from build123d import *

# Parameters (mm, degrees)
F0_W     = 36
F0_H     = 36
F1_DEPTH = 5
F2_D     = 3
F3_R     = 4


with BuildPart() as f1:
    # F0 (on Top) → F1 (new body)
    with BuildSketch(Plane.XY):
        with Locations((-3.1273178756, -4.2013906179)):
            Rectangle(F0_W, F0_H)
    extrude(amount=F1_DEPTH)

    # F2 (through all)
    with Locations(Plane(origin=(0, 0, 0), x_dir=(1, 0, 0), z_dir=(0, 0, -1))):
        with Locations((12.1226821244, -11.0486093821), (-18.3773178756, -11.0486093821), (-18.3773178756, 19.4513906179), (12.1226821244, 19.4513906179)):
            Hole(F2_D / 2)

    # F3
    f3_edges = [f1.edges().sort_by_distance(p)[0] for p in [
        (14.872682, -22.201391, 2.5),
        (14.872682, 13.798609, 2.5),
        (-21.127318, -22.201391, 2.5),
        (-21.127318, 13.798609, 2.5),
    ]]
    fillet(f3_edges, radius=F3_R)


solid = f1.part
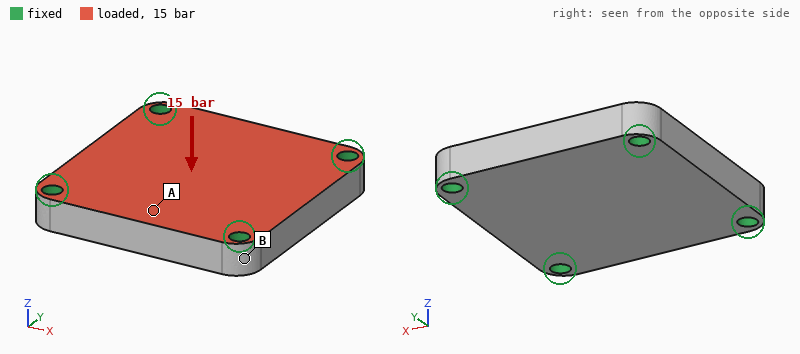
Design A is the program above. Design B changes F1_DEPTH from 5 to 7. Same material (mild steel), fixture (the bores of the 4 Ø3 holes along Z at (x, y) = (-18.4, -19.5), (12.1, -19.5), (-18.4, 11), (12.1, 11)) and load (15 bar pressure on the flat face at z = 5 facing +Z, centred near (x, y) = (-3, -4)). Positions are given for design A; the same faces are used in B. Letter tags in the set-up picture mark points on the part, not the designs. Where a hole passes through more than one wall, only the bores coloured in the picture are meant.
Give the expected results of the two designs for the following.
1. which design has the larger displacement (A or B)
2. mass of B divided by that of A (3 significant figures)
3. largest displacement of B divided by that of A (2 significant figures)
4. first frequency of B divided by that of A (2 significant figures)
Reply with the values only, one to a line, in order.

A
1.40
0.44
1.3
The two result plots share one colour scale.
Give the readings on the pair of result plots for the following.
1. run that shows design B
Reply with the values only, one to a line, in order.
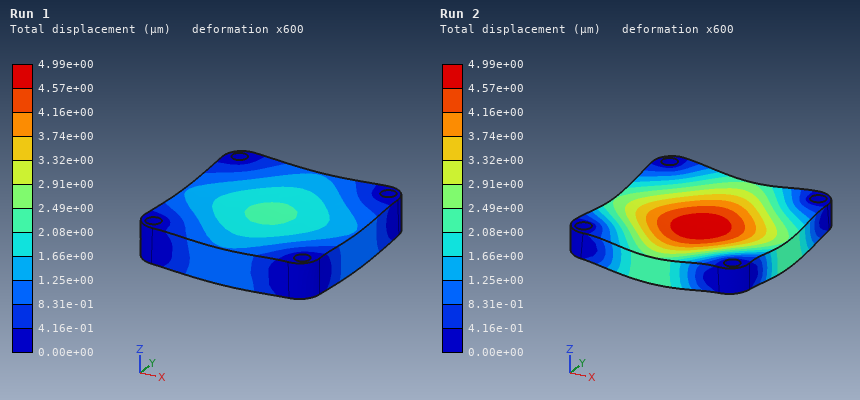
Run 1
